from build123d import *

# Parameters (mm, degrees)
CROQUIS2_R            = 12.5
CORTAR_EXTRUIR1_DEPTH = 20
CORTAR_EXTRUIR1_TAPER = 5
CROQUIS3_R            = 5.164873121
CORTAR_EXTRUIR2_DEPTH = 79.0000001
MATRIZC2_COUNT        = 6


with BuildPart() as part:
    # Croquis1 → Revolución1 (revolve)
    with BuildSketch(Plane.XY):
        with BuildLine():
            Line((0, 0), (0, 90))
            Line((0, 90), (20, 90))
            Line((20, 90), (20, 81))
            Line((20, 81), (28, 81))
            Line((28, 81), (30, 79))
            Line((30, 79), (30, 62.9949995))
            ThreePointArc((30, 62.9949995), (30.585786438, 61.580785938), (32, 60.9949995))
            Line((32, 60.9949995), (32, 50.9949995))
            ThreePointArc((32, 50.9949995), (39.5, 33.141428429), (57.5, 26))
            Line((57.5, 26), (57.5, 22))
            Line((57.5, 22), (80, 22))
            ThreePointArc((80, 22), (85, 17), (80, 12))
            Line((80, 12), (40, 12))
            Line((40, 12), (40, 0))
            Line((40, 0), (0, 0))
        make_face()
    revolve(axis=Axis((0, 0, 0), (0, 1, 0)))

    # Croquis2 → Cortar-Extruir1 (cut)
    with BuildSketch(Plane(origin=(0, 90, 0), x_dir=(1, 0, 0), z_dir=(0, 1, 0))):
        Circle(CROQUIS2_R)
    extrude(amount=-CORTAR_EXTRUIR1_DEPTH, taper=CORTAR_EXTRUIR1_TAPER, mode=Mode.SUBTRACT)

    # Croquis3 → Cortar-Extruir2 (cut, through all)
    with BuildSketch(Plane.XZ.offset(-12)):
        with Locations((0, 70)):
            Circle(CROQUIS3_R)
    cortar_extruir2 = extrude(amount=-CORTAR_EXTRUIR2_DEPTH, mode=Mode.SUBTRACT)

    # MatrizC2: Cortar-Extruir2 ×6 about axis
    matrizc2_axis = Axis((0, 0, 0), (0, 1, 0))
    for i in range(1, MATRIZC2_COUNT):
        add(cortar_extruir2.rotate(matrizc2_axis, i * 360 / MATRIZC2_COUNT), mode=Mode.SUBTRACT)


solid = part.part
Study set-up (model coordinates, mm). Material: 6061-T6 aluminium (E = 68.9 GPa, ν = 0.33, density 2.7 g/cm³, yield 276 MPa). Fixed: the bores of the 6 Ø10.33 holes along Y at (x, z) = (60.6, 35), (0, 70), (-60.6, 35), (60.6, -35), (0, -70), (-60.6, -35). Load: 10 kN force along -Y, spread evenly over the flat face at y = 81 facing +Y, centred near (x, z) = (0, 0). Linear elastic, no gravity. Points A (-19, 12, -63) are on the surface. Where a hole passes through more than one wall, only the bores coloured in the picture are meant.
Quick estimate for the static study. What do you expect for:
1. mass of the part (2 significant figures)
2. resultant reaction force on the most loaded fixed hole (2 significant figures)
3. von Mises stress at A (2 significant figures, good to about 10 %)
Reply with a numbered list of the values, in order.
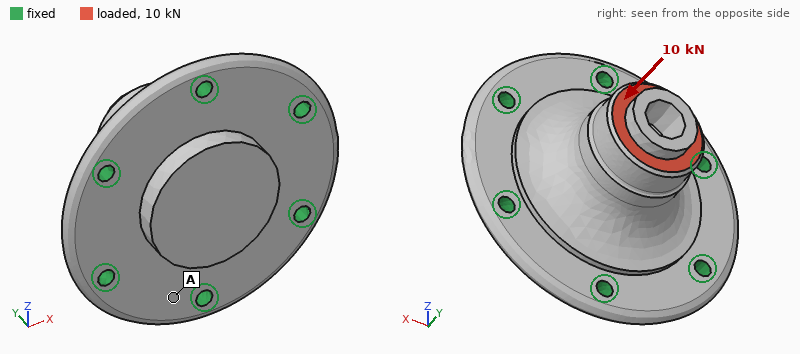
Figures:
1. 1.4 kg
2. 1.9 kN
3. 3.9 MPa
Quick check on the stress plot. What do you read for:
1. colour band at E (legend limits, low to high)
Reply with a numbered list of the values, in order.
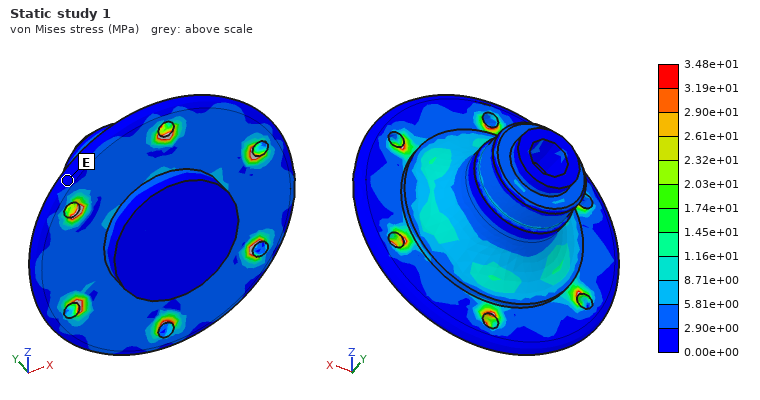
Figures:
1. 0.00e+00 to 2.90e+00 MPa
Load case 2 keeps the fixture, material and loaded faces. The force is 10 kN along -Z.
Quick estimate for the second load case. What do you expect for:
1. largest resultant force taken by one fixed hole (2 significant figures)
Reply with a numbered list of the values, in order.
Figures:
1. 4.4 kN
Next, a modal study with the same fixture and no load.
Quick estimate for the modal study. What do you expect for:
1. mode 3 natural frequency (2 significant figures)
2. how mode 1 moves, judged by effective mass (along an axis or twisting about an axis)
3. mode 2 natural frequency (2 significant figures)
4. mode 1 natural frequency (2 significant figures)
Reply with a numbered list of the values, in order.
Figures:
1. 5400 Hz
2. along Y
3. 5400 Hz
4. 4500 Hz
